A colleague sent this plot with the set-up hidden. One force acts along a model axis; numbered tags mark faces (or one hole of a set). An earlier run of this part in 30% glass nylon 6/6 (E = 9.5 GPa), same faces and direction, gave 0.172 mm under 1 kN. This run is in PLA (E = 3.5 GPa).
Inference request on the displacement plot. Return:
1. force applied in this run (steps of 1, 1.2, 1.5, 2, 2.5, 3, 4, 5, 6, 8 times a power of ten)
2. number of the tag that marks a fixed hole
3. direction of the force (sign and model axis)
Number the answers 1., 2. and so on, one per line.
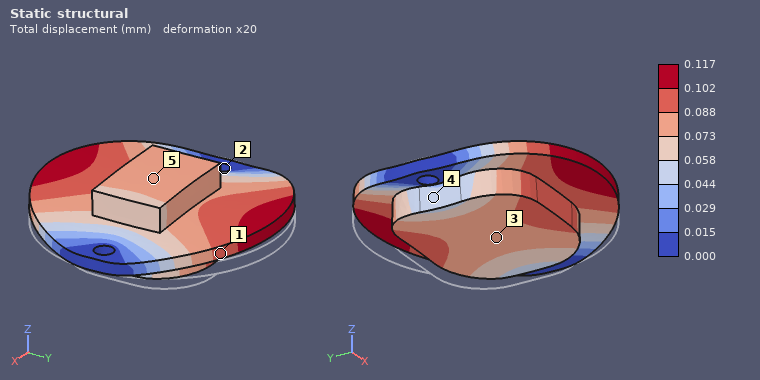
1. 250 N
2. 2
3. +Z
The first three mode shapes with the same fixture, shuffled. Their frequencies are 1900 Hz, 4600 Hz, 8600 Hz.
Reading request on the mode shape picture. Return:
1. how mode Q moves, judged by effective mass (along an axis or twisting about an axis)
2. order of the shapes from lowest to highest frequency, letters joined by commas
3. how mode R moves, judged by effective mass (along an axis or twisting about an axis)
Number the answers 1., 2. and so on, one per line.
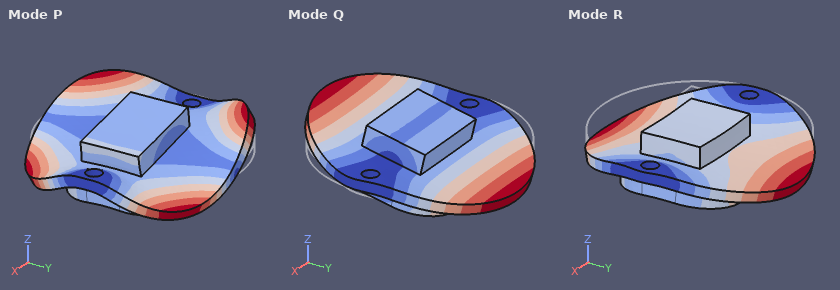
1. twisting about X
2. Q, R, P
3. along Z
